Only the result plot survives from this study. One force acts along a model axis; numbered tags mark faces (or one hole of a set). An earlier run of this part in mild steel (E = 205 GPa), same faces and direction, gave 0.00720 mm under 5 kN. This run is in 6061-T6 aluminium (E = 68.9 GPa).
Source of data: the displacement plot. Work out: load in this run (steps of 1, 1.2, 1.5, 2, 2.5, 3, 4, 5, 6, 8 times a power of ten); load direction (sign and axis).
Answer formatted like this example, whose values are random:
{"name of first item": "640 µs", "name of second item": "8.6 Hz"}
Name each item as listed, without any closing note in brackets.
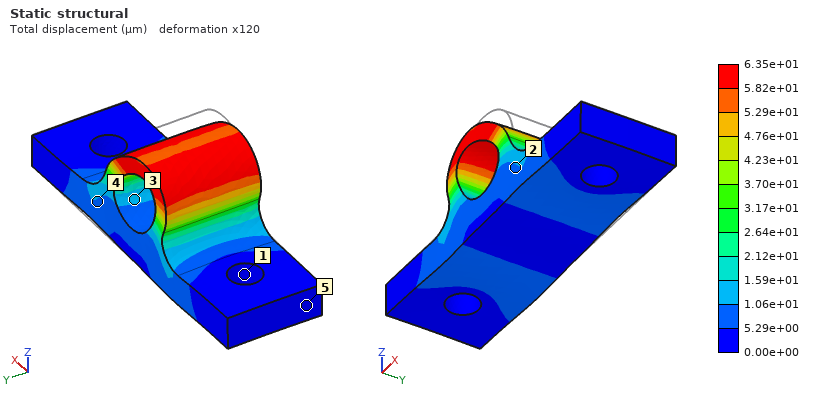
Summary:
{"load in this run": "15 kN", "load direction": "-X"}
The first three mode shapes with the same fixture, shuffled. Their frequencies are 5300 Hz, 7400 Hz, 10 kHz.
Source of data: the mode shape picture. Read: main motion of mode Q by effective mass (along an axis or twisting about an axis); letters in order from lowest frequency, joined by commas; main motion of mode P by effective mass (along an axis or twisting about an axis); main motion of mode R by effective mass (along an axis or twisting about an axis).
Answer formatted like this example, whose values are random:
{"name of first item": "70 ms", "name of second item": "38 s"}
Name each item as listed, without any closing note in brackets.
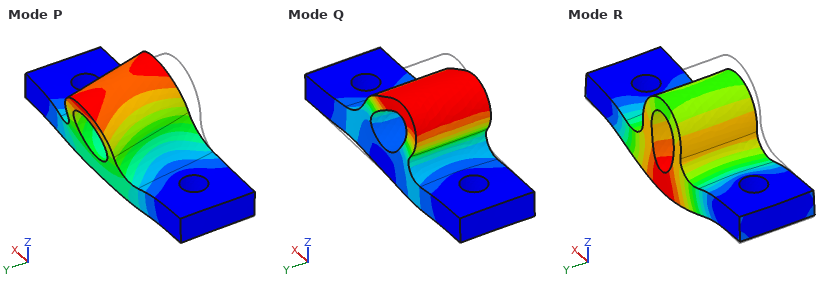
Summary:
{"main motion of mode Q by effective mass": "along X", "letters in order from lowest frequency, joined by commas": "P, R, Q", "main motion of mode P by effective mass": "along Y", "main motion of mode R by effective mass": "along Z"}
